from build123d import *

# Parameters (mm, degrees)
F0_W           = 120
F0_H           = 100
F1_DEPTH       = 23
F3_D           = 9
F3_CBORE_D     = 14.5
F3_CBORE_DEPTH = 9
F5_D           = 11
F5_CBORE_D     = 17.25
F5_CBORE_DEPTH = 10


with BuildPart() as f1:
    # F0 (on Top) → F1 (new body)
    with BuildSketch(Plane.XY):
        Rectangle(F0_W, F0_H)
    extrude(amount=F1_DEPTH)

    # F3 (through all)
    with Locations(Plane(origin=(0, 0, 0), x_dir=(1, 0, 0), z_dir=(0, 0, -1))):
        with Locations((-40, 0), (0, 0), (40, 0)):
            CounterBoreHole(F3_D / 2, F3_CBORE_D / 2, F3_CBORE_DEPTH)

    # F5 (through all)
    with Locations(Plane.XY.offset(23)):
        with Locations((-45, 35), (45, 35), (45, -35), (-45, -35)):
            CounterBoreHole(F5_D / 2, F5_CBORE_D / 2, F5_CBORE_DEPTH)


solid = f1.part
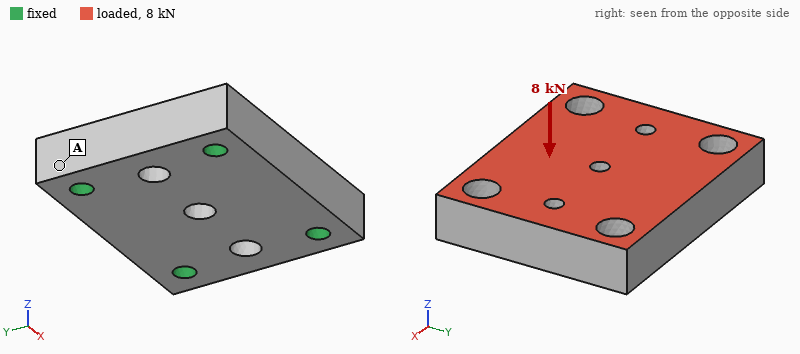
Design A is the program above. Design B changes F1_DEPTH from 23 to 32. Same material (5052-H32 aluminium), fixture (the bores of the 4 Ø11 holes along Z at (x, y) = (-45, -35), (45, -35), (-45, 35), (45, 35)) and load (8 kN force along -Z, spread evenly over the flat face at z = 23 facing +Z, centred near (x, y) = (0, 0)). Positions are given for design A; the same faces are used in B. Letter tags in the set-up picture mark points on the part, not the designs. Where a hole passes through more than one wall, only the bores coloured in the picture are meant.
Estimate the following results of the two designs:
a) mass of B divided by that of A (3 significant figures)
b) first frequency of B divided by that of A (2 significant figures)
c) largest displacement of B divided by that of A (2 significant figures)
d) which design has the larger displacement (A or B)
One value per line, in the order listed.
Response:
1.38
1.1
0.58
A
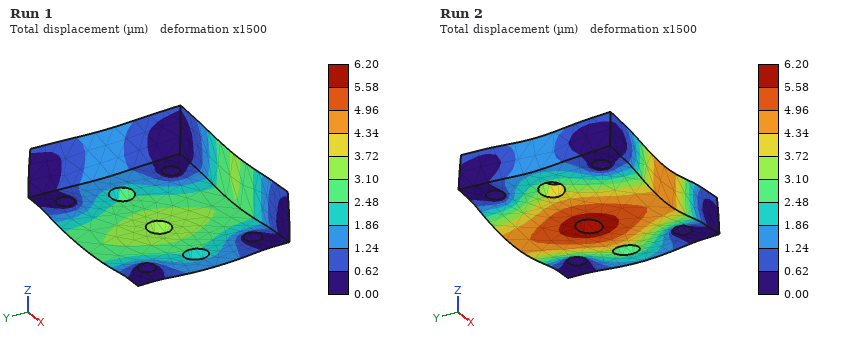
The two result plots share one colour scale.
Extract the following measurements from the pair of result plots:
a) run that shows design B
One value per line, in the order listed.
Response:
Run 1
